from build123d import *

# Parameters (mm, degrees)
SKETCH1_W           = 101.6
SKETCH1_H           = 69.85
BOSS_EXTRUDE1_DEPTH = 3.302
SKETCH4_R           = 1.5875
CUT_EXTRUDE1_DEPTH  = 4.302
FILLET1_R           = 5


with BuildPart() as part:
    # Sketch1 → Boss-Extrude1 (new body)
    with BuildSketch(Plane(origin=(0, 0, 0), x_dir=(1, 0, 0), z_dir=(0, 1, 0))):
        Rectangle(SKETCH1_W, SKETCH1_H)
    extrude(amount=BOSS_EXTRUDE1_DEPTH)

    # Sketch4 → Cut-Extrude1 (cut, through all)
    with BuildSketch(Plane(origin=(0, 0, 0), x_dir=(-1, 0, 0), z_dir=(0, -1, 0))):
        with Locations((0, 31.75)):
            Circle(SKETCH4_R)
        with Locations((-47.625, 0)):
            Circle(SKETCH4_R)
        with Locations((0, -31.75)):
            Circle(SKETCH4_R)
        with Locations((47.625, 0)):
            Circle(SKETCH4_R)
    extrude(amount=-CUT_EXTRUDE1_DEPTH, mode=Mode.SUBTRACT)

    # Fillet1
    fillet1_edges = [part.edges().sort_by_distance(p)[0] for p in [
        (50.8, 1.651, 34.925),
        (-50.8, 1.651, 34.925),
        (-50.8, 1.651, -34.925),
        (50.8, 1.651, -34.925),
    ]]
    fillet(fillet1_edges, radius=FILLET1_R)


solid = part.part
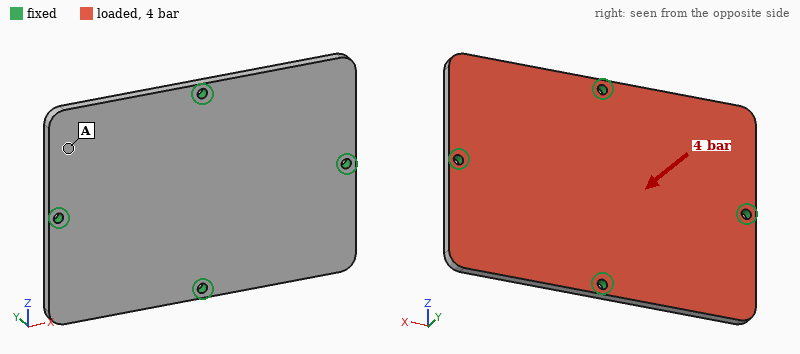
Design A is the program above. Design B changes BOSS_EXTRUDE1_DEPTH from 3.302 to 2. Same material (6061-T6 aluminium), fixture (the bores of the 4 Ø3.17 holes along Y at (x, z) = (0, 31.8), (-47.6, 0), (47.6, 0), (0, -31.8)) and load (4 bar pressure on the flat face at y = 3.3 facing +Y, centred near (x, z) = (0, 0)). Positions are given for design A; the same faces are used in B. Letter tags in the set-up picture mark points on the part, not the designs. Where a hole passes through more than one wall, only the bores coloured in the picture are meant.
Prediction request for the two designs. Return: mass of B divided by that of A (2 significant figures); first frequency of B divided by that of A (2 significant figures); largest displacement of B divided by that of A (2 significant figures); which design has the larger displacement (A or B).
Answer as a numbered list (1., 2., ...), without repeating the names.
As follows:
1. 0.61
2. 0.63
3. 4.4
4. B
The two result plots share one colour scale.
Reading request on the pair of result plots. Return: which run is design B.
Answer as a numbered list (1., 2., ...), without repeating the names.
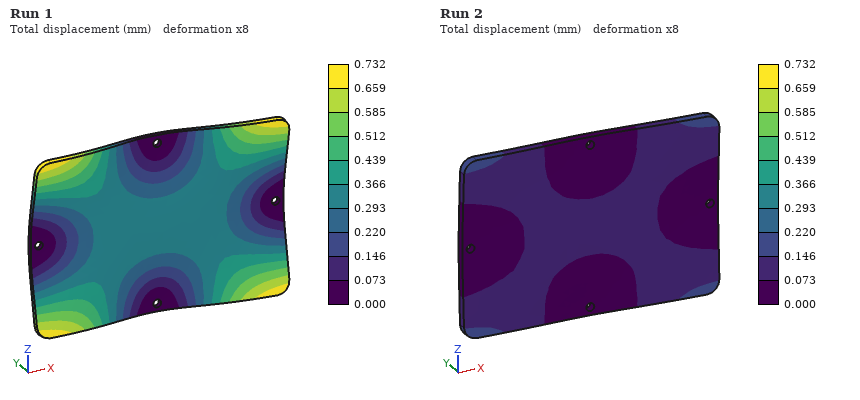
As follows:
1. Run 1
